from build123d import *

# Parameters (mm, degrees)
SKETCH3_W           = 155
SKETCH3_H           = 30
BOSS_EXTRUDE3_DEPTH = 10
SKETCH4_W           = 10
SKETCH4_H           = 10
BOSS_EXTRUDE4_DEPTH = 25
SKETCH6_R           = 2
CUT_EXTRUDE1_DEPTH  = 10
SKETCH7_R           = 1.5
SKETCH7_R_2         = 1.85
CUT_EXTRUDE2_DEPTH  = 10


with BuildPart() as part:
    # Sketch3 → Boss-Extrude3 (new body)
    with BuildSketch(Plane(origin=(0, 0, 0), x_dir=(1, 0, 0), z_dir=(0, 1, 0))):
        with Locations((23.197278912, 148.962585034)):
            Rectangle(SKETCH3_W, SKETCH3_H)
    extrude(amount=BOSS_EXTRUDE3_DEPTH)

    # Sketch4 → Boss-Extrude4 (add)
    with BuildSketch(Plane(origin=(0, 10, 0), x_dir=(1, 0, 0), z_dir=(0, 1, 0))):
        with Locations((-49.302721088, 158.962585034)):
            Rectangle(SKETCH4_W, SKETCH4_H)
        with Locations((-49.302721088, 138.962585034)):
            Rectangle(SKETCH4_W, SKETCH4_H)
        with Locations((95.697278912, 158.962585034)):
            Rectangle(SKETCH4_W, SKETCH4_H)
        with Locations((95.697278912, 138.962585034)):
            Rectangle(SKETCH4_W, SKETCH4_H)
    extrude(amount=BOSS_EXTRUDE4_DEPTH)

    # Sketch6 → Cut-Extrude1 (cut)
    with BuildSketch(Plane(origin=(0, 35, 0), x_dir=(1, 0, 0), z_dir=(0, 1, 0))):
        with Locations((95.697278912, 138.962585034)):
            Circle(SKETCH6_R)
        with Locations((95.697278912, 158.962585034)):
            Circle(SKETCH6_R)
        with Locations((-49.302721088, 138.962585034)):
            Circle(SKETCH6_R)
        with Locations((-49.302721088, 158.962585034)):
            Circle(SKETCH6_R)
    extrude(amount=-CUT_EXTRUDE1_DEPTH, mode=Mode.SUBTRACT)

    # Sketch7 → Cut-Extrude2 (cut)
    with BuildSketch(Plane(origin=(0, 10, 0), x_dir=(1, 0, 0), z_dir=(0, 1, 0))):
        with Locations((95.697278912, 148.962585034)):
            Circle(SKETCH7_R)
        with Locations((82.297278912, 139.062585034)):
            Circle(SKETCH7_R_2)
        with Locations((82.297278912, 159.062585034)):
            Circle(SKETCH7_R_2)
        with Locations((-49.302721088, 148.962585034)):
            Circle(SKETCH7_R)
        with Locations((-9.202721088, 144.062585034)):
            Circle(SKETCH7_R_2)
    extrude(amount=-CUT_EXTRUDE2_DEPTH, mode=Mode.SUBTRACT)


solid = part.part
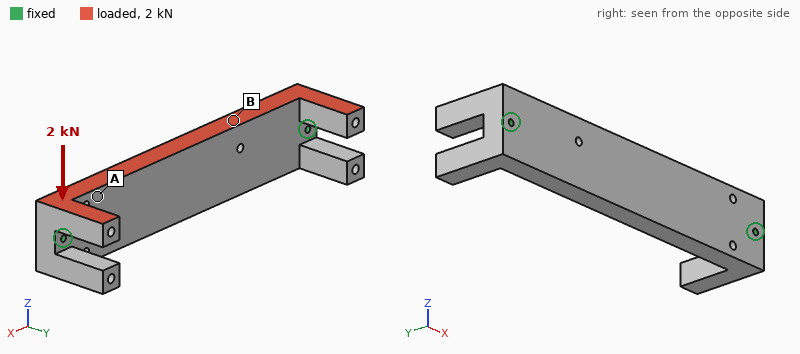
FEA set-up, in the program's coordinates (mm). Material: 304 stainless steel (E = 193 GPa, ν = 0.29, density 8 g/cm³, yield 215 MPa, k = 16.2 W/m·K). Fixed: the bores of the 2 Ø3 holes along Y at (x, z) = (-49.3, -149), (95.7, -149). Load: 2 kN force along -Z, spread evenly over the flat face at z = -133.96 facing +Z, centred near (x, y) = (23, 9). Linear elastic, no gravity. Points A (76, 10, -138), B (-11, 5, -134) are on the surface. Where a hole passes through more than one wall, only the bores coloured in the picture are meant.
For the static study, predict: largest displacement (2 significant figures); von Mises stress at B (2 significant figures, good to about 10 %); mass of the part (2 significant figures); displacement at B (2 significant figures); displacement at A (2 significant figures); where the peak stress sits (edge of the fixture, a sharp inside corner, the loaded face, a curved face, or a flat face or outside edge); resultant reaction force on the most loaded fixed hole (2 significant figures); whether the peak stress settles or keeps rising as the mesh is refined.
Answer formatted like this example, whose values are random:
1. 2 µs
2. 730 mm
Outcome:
1. 12 µm
2. 10 MPa
3. 440 g
4. 8.9 µm
5. 6.0 µm
6. edge of the fixture
7. 1.0 kN
8. keeps rising
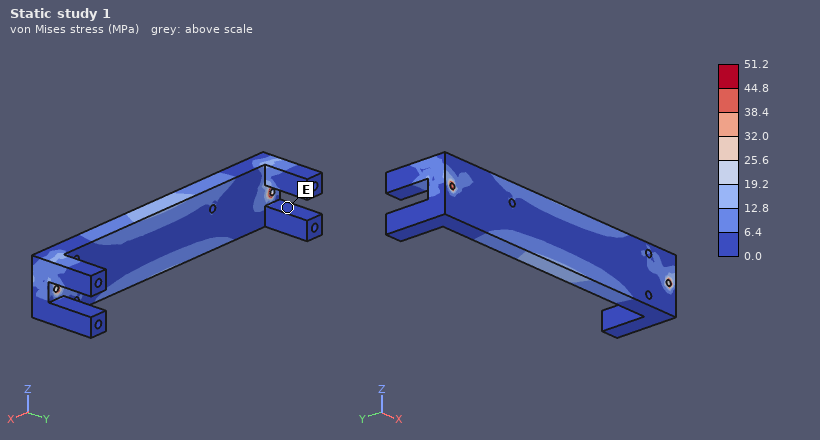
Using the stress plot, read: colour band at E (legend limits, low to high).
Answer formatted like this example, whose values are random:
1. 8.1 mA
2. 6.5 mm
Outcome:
1. 0.0 to 6.4 MPa
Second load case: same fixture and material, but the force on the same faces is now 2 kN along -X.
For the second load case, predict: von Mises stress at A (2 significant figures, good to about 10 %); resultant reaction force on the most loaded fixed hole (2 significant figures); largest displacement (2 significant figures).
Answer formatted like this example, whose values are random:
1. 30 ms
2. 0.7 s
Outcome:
1. 3.8 MPa
2. 1.0 kN
3. 11 µm
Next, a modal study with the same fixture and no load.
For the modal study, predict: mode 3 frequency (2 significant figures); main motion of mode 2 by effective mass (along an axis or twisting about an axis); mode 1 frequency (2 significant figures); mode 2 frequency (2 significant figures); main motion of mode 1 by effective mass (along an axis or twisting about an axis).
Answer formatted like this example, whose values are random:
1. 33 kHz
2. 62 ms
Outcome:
1. 4800 Hz
2. along Z
3. 2000 Hz
4. 3300 Hz
5. along Y
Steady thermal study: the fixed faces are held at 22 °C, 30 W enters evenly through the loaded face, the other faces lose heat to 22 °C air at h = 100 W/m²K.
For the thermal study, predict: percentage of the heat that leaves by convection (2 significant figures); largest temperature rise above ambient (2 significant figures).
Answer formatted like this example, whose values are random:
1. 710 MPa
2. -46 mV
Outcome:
1. 71 %
2. 29 K
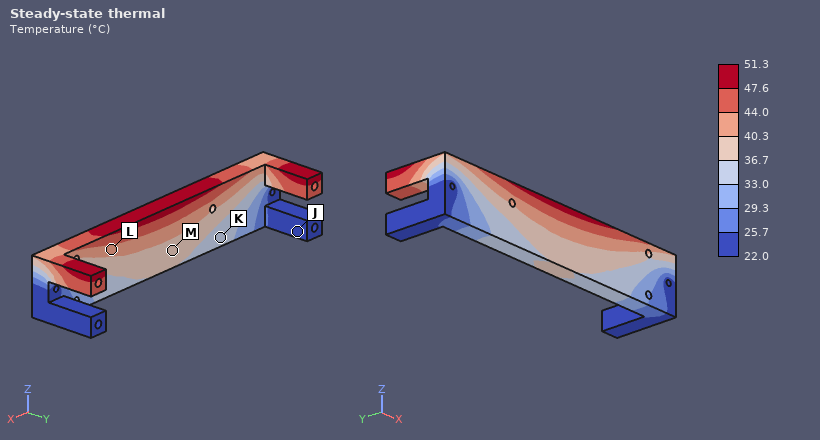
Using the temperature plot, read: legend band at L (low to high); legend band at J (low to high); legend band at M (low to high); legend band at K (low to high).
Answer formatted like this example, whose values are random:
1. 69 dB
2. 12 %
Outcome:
1. 40.3 to 44.0 °C
2. 22.0 to 25.7 °C
3. 36.7 to 40.3 °C
4. 33.0 to 36.7 °C
